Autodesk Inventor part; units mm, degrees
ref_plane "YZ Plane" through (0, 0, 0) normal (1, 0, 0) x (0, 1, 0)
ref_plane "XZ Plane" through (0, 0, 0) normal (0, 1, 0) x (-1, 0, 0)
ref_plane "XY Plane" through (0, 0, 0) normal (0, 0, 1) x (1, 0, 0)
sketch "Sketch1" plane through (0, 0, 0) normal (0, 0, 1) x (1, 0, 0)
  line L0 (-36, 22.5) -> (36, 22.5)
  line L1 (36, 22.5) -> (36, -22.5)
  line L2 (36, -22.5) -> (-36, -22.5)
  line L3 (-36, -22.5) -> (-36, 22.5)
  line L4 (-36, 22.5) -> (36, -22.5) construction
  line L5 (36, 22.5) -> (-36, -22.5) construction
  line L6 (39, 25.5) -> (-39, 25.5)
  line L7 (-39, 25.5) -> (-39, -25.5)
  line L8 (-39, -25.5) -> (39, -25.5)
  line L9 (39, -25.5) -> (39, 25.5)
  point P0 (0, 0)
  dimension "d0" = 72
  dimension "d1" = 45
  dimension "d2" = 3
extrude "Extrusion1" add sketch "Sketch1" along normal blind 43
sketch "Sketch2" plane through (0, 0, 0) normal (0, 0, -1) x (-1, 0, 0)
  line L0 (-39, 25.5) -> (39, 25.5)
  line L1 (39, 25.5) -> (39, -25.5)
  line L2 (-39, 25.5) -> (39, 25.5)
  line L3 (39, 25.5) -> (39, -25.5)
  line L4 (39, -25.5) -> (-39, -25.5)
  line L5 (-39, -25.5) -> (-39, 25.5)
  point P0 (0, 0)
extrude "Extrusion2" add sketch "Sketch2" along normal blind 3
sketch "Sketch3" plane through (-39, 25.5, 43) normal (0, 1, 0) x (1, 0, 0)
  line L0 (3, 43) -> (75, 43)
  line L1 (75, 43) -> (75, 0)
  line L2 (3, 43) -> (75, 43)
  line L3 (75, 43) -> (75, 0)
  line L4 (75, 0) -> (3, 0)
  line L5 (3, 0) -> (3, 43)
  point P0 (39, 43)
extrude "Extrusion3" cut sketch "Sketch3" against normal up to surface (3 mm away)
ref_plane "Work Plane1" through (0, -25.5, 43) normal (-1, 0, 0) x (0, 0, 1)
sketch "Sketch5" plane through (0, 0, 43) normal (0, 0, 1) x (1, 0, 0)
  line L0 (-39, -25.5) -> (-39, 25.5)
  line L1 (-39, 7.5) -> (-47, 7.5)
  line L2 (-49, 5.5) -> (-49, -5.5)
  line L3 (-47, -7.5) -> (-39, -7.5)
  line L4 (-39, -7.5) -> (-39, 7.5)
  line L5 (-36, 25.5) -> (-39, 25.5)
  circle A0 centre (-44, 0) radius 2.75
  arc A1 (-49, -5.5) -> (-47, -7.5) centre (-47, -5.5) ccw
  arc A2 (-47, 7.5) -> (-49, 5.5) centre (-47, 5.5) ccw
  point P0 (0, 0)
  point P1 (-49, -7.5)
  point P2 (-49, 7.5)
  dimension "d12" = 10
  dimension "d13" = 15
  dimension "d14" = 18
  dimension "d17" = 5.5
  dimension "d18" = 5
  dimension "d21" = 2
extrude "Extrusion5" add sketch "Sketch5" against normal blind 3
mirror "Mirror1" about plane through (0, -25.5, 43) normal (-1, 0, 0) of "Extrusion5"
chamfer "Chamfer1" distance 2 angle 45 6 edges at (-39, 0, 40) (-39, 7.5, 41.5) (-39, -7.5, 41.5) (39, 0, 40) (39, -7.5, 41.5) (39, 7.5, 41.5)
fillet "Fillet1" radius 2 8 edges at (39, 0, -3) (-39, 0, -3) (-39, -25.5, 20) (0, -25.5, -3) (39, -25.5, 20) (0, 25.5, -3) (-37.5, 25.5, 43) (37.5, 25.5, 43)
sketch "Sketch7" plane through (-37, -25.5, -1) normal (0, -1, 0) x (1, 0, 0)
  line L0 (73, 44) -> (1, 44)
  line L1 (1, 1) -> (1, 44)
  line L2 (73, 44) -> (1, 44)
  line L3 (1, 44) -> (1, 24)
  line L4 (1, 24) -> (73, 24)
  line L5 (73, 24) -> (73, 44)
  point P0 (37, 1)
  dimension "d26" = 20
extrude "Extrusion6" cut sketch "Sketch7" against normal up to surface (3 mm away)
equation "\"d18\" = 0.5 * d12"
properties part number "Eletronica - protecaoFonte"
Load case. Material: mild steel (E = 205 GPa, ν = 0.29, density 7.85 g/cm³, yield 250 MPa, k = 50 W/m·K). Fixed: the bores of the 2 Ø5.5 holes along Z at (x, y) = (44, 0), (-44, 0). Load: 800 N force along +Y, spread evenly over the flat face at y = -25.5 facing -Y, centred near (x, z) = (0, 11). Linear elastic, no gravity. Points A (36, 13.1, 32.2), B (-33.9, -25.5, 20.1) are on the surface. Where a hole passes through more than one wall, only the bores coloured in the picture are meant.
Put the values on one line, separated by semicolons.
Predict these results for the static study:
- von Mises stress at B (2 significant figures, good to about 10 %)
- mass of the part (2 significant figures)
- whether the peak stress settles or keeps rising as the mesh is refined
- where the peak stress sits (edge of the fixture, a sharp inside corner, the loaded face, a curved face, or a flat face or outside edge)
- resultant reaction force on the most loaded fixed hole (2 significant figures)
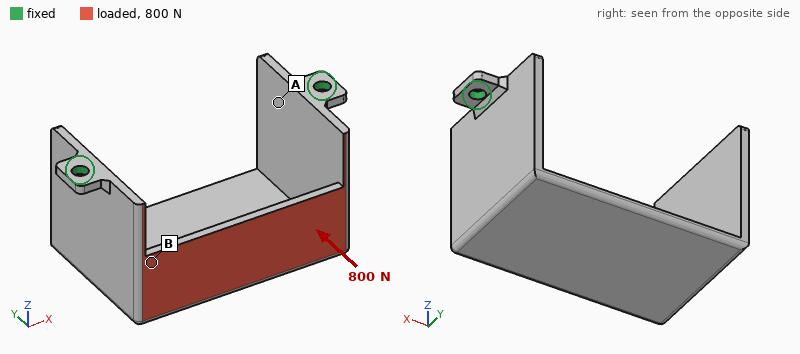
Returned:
38 MPa; 240 g; keeps rising; edge of the fixture; 400 N
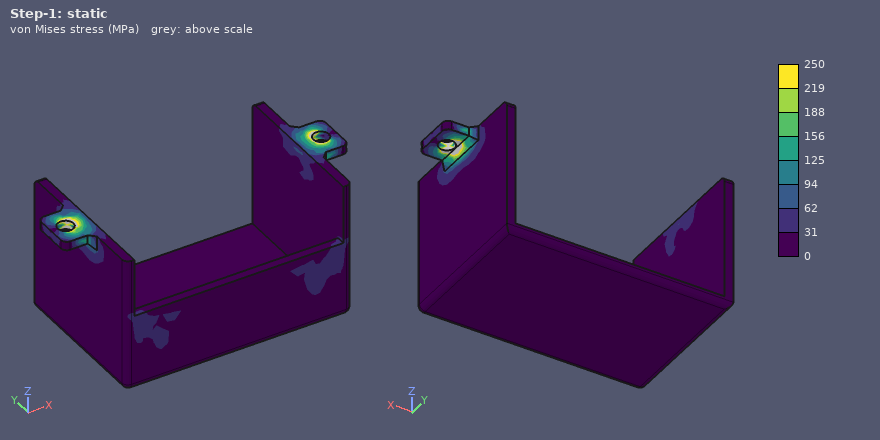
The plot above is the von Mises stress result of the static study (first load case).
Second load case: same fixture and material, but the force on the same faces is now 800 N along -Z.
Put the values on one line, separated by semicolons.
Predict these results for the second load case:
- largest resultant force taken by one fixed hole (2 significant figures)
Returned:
410 N
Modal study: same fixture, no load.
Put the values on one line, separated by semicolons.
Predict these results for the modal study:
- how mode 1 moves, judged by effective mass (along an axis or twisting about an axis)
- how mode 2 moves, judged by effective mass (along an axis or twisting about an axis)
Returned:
along Y; along X
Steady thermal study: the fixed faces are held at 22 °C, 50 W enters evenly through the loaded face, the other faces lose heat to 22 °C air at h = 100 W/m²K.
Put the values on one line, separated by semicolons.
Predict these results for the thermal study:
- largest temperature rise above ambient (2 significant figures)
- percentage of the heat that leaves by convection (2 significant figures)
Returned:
79 K; 90 %
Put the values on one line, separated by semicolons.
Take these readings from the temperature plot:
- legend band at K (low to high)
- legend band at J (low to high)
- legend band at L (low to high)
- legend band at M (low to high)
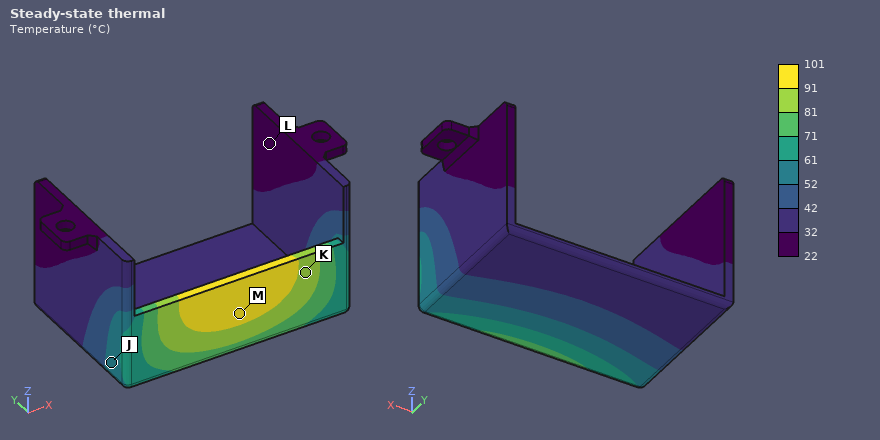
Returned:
81 to 91 °C; 52 to 61 °C; 22 to 32 °C; 91 to 101 °C
